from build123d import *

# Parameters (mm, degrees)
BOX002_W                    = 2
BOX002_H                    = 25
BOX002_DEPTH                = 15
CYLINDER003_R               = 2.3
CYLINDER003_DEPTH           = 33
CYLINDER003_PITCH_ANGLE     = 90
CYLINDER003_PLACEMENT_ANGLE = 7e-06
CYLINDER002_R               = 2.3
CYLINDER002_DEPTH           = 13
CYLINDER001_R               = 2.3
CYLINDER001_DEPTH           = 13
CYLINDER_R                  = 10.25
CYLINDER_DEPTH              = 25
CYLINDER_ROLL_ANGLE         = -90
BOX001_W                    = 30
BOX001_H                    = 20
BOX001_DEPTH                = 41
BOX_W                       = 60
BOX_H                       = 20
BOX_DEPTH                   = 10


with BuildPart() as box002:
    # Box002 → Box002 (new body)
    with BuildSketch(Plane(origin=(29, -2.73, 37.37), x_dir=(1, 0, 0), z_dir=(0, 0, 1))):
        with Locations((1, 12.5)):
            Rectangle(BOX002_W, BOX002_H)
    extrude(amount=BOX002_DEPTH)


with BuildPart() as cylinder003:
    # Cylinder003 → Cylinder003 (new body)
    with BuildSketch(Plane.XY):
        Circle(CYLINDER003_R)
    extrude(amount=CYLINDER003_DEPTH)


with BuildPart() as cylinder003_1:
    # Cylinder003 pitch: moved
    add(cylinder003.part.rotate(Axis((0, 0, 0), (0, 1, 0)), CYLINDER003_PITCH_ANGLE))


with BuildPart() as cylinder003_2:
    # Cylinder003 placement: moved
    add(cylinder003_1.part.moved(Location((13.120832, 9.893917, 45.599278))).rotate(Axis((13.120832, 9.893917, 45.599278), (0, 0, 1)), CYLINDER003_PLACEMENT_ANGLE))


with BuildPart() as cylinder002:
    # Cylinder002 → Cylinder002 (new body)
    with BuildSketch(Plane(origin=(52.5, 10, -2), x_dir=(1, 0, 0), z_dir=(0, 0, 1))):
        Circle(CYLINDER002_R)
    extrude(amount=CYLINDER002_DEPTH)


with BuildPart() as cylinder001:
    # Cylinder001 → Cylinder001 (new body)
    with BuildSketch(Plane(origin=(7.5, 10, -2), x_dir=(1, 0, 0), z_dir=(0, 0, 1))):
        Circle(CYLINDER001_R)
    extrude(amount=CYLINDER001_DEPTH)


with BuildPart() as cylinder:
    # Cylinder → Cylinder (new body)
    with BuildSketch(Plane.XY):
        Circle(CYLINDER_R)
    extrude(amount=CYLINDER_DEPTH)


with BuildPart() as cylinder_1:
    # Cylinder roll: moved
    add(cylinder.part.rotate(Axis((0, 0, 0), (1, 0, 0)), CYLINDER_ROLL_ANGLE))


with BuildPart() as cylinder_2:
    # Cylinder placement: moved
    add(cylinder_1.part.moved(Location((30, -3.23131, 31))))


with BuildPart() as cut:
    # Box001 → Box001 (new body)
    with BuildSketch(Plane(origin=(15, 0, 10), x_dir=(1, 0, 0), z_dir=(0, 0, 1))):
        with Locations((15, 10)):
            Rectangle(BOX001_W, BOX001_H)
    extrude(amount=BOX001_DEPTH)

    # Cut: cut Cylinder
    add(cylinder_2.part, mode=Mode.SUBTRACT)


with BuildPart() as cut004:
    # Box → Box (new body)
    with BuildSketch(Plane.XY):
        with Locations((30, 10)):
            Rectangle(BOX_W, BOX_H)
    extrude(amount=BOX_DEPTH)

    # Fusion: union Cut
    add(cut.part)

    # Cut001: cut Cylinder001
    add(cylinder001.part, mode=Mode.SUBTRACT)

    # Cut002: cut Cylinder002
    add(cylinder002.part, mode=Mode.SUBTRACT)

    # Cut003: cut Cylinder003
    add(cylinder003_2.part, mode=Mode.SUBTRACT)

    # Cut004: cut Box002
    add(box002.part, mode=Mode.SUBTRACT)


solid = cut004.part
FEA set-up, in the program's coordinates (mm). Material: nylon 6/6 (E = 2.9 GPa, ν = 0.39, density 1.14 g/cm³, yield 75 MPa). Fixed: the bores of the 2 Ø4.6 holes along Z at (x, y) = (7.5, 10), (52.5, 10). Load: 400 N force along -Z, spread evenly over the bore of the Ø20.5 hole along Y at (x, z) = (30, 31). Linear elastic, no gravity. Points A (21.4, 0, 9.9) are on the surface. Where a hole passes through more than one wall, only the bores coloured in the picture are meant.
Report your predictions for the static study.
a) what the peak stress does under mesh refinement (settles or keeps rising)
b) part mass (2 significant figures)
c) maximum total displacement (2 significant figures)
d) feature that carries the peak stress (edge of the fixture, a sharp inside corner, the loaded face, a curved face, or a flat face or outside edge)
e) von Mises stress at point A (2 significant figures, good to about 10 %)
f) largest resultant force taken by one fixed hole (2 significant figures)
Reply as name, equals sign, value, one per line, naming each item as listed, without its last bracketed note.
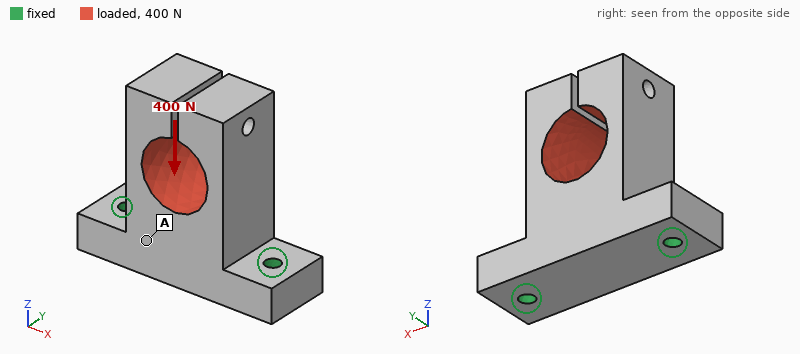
what the peak stress does under mesh refinement = keeps rising
part mass = 33 g
maximum total displacement = 0.29 mm
feature that carries the peak stress = edge of the fixture
von Mises stress at point A = 1.00 MPa
largest resultant force taken by one fixed hole = 210 N
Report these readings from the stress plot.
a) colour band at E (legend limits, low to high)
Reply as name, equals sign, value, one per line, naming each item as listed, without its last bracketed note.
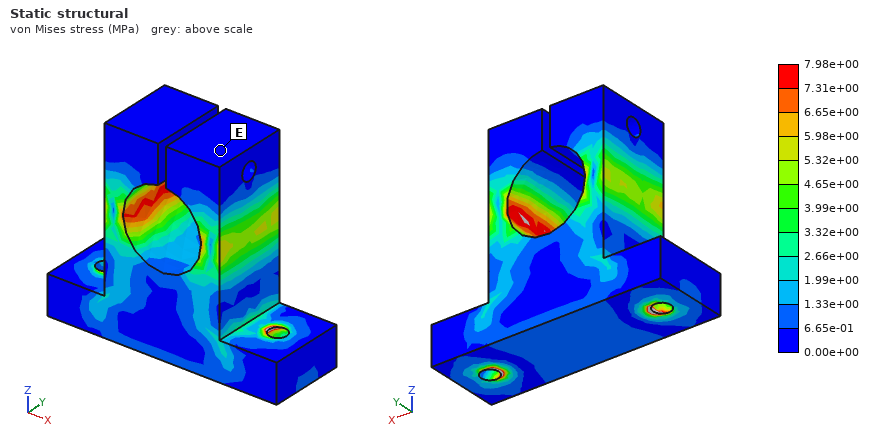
colour band at E = 0.00e+00 to 6.65e-01 MPa
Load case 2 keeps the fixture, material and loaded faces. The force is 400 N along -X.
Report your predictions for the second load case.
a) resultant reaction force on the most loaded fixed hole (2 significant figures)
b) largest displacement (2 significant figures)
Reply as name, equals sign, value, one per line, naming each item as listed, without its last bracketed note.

resultant reaction force on the most loaded fixed hole = 330 N
largest displacement = 0.52 mm
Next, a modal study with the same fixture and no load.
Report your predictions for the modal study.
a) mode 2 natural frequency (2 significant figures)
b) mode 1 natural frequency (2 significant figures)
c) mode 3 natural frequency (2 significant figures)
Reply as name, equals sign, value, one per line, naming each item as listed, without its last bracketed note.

mode 2 natural frequency = 1000 Hz
mode 1 natural frequency = 1000 Hz
mode 3 natural frequency = 1000 Hz
